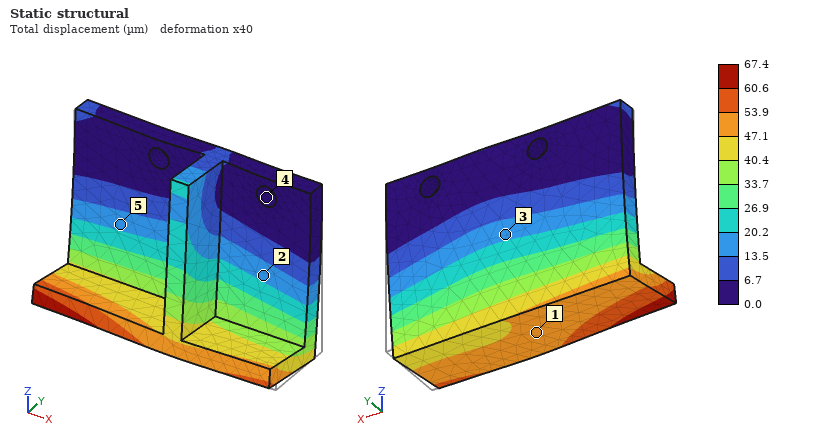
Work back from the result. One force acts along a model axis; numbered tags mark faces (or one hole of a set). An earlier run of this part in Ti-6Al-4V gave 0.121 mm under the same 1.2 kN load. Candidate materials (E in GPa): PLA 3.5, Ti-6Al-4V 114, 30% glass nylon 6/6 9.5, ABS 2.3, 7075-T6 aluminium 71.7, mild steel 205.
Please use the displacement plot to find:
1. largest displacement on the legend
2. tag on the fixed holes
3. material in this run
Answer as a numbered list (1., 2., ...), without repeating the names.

1. 67.4 µm
2. 4
3. mild steel
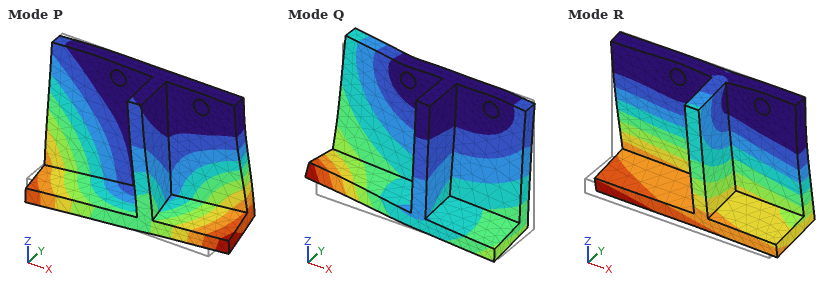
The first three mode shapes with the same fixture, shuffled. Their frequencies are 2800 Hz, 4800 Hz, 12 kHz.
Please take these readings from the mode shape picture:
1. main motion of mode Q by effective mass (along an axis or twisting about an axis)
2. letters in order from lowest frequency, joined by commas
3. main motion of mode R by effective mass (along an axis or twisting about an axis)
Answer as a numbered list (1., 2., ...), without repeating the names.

1. along X
2. R, P, Q
3. along Y
